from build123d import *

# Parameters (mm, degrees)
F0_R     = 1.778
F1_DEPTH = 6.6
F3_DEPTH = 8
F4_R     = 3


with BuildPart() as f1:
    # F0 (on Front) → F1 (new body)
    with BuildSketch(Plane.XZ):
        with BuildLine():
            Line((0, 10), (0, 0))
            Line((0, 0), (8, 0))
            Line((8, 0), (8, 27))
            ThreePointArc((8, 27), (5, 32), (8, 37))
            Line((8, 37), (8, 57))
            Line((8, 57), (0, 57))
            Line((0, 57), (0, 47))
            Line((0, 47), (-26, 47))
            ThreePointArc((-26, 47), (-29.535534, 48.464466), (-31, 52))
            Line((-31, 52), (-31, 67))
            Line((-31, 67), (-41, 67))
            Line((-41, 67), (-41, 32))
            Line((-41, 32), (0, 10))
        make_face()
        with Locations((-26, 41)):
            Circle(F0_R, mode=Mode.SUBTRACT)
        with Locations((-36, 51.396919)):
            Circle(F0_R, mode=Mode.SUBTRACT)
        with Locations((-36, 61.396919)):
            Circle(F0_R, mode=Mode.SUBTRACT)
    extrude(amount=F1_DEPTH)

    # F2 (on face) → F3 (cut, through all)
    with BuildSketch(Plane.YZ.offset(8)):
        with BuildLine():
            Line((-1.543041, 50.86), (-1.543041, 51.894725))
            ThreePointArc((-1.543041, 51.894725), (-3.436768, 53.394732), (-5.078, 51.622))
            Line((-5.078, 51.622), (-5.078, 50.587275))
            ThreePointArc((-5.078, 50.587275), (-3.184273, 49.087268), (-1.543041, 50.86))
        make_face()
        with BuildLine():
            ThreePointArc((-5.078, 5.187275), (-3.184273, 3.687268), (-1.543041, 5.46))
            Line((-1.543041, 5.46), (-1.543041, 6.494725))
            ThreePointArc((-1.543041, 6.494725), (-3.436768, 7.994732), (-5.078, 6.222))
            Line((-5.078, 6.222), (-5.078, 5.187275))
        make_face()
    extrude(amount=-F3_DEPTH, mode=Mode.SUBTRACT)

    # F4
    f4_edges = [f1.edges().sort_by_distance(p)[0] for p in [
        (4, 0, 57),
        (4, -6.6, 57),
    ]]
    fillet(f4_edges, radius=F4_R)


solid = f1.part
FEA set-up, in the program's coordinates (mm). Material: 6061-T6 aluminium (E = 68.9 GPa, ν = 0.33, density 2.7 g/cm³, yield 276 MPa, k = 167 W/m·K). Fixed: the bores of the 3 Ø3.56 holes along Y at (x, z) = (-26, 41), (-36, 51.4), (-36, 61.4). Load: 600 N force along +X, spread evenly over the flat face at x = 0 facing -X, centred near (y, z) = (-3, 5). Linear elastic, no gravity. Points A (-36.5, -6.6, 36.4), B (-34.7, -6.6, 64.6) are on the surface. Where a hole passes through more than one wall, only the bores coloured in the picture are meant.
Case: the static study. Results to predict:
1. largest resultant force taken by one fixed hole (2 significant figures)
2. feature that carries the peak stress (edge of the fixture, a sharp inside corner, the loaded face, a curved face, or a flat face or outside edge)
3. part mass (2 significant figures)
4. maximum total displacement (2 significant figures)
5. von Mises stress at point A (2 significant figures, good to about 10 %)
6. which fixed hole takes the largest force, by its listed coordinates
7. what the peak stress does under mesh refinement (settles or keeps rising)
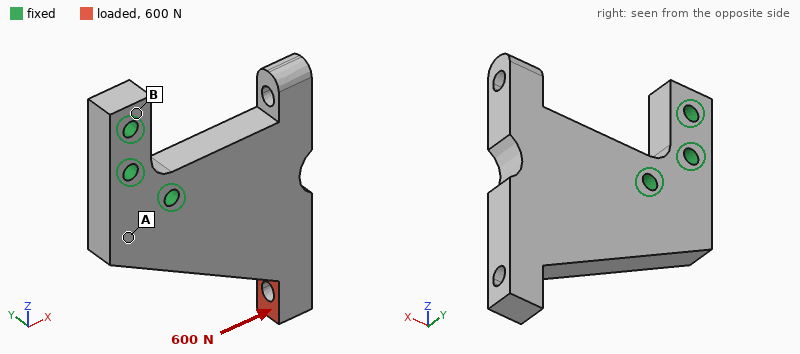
1.5 kN
edge of the fixture
29 g
0.11 mm
25 MPa
(-26, 41)
keeps rising
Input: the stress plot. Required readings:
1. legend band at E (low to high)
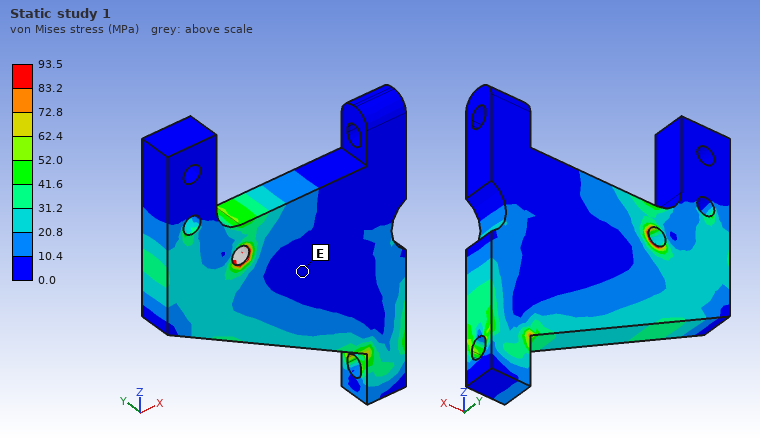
0.0 to 10.4 MPa
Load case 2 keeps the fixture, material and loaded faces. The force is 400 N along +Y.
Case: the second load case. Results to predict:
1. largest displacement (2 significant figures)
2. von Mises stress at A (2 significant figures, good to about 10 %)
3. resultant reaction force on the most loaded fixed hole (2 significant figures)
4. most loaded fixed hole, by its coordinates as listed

0.45 mm
35 MPa
770 N
(-26, 41)
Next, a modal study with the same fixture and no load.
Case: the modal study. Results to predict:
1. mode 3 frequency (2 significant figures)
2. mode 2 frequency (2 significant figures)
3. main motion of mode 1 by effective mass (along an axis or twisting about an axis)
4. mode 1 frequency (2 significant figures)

4900 Hz
4800 Hz
along Y
2600 Hz
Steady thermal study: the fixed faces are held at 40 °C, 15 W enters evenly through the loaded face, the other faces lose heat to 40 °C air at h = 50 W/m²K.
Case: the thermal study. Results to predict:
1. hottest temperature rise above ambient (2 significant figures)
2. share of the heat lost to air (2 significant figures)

46 K
16 %
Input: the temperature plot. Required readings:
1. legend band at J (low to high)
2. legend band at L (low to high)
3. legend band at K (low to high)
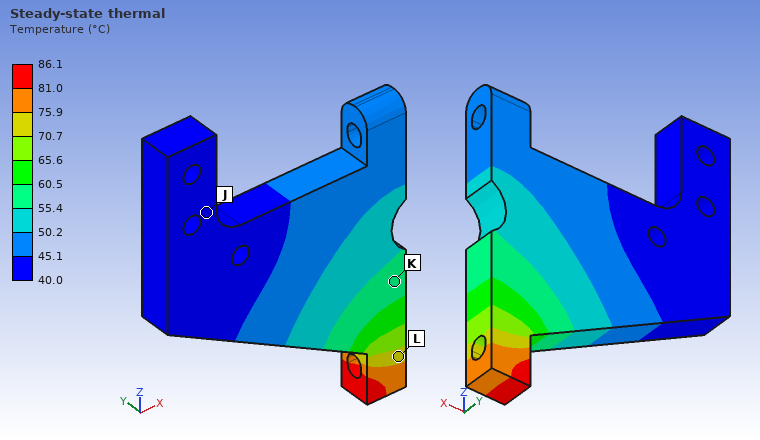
40.0 to 45.1 °C
70.7 to 75.9 °C
55.4 to 60.5 °C
